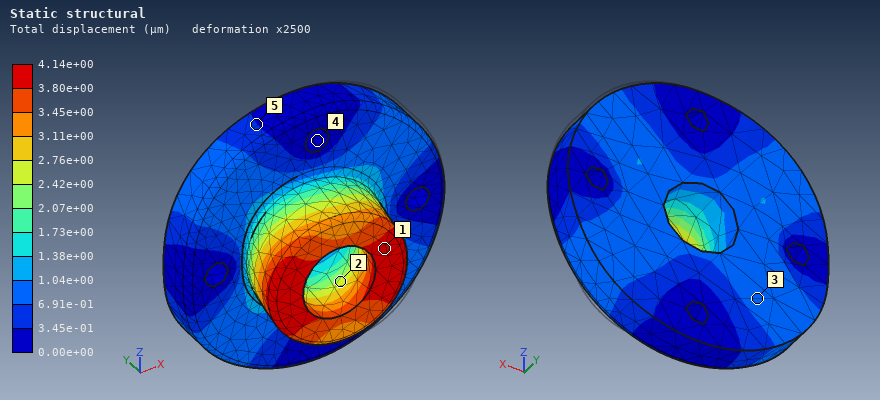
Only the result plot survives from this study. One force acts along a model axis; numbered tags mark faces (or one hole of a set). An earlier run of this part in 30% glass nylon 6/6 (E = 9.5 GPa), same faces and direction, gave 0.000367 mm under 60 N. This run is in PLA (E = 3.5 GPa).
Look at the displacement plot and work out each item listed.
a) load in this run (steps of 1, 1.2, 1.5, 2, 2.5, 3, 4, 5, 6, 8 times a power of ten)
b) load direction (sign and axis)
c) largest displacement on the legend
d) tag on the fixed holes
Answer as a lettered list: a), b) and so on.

a) 250 N
b) -X
c) 4.14e+00 µm
d) 4
